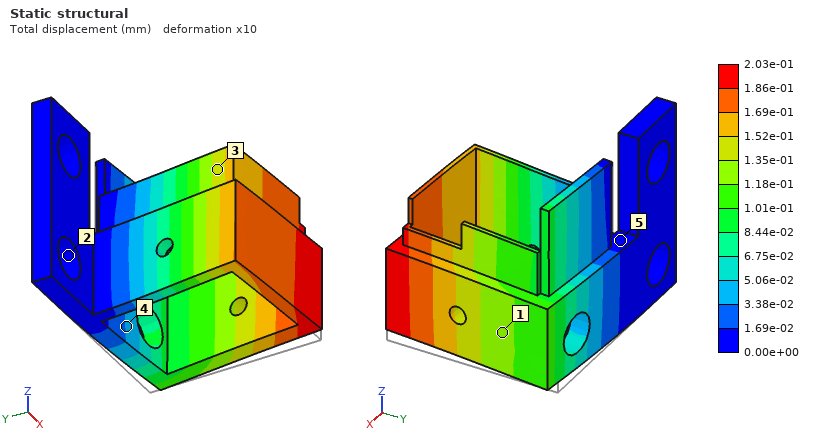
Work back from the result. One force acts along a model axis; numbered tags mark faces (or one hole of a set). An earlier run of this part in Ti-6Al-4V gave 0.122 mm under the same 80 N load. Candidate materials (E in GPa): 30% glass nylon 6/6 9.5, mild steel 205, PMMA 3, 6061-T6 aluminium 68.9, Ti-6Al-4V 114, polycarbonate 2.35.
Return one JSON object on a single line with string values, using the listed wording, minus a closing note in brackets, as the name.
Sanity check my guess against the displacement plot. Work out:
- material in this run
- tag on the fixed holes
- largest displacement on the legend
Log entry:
{"material in this run": "6061-T6 aluminium", "tag on the fixed holes": "2", "largest displacement on the legend": "2.03e-01 mm"}
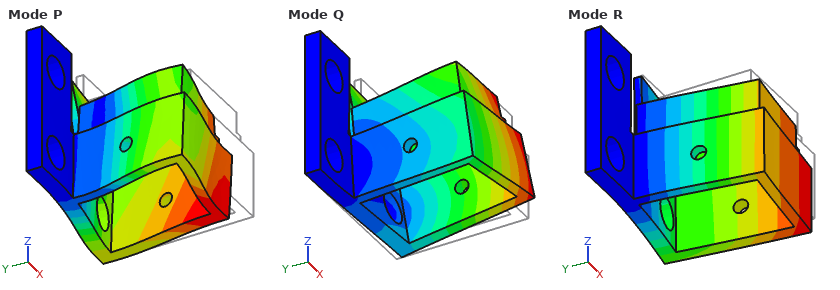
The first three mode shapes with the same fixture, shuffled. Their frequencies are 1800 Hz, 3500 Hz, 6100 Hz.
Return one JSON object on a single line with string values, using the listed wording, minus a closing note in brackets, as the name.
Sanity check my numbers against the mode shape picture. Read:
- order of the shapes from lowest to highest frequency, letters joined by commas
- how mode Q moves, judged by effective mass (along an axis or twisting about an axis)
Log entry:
{"order of the shapes from lowest to highest frequency, letters joined by commas": "R, Q, P", "how mode Q moves, judged by effective mass": "along Z"}
